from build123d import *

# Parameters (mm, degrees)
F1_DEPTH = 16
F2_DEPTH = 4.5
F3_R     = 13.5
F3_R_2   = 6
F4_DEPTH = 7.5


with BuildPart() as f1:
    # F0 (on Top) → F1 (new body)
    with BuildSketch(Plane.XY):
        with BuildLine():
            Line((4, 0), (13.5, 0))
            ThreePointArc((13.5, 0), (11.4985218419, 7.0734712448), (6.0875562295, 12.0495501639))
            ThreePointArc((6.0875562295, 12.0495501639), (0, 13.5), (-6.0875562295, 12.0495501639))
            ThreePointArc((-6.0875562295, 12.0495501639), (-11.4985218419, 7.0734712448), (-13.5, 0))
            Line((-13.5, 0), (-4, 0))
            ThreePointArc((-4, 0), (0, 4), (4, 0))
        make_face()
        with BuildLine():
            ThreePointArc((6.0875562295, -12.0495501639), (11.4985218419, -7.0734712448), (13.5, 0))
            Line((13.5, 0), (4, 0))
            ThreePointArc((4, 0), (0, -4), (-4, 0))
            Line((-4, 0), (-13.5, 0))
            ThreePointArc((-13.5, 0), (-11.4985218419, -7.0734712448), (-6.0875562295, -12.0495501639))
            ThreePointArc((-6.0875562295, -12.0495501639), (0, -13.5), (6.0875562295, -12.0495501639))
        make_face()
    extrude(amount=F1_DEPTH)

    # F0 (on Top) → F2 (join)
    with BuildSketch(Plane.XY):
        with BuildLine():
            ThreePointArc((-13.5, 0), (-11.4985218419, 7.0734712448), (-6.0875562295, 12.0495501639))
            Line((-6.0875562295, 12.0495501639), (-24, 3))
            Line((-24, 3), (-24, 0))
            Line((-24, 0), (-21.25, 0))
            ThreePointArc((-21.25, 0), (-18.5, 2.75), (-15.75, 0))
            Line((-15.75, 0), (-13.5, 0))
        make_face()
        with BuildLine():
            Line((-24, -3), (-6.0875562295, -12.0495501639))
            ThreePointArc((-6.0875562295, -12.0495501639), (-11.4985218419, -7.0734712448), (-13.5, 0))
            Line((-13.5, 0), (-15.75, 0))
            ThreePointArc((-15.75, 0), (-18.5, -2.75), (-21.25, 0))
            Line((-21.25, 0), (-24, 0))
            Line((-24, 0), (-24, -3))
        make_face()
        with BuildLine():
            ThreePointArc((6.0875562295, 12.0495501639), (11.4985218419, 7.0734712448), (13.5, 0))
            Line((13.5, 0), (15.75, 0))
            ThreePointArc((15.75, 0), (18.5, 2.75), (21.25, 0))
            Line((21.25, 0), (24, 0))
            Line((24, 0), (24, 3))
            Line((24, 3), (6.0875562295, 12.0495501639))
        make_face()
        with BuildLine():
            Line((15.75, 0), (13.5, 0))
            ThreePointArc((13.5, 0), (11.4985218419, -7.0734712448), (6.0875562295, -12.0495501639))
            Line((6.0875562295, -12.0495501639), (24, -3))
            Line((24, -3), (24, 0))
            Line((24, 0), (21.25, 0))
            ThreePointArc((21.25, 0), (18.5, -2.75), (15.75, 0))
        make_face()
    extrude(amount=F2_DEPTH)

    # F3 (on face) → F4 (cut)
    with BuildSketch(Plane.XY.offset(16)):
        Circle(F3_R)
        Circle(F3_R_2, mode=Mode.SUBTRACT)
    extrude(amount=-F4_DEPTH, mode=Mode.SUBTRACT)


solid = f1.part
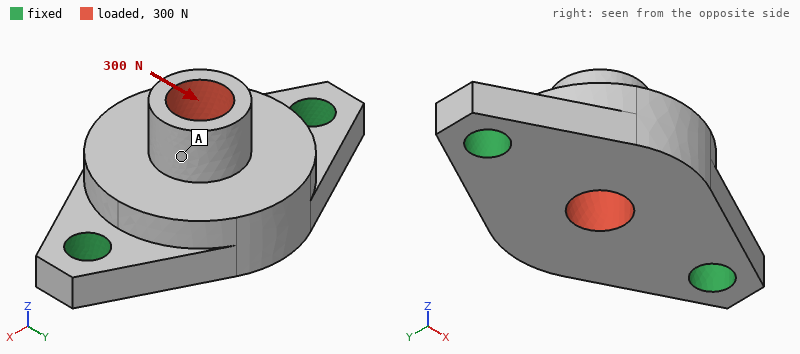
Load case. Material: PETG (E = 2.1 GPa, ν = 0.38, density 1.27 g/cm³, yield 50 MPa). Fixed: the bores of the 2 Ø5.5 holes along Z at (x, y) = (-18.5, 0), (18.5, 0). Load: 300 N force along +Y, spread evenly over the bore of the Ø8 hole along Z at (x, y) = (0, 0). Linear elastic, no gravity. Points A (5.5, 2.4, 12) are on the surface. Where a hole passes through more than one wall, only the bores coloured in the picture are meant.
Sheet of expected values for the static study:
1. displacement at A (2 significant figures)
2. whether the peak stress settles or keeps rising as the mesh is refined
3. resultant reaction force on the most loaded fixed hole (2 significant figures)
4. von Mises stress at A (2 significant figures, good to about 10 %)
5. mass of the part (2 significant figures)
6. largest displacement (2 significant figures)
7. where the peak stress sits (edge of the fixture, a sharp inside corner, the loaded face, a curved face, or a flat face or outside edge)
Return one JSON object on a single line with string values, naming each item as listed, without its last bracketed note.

{"displacement at A": "0.19 mm", "whether the peak stress settles or keeps rising as the mesh is refined": "keeps rising", "resultant reaction force on the most loaded fixed hole": "150 N", "von Mises stress at A": "2.7 MPa", "mass of the part": "7.6 g", "largest displacement": "0.27 mm", "where the peak stress sits": "edge of the fixture"}
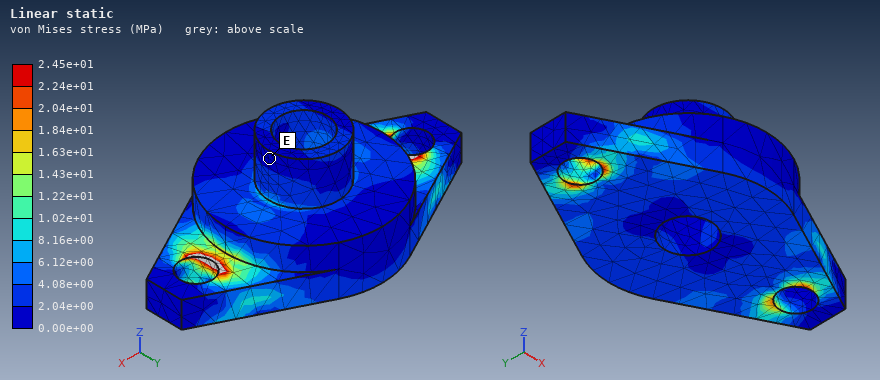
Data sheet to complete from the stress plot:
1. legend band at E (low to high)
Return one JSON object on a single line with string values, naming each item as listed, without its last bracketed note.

{"legend band at E": "0.00e+00 to 2.04e+00 MPa"}
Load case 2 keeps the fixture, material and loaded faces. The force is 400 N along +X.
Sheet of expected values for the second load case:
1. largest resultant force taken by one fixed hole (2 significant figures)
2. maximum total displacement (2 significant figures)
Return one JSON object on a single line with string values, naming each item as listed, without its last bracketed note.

{"largest resultant force taken by one fixed hole": "210 N", "maximum total displacement": "81 µm"}
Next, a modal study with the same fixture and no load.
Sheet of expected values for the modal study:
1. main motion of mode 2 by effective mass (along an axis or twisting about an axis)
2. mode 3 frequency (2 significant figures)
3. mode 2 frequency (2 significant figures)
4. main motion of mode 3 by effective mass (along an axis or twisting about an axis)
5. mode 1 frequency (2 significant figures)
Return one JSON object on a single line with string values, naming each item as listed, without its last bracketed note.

{"main motion of mode 2 by effective mass": "along Z", "mode 3 frequency": "6900 Hz", "mode 2 frequency": "4200 Hz", "main motion of mode 3 by effective mass": "along Y", "mode 1 frequency": "2700 Hz"}
